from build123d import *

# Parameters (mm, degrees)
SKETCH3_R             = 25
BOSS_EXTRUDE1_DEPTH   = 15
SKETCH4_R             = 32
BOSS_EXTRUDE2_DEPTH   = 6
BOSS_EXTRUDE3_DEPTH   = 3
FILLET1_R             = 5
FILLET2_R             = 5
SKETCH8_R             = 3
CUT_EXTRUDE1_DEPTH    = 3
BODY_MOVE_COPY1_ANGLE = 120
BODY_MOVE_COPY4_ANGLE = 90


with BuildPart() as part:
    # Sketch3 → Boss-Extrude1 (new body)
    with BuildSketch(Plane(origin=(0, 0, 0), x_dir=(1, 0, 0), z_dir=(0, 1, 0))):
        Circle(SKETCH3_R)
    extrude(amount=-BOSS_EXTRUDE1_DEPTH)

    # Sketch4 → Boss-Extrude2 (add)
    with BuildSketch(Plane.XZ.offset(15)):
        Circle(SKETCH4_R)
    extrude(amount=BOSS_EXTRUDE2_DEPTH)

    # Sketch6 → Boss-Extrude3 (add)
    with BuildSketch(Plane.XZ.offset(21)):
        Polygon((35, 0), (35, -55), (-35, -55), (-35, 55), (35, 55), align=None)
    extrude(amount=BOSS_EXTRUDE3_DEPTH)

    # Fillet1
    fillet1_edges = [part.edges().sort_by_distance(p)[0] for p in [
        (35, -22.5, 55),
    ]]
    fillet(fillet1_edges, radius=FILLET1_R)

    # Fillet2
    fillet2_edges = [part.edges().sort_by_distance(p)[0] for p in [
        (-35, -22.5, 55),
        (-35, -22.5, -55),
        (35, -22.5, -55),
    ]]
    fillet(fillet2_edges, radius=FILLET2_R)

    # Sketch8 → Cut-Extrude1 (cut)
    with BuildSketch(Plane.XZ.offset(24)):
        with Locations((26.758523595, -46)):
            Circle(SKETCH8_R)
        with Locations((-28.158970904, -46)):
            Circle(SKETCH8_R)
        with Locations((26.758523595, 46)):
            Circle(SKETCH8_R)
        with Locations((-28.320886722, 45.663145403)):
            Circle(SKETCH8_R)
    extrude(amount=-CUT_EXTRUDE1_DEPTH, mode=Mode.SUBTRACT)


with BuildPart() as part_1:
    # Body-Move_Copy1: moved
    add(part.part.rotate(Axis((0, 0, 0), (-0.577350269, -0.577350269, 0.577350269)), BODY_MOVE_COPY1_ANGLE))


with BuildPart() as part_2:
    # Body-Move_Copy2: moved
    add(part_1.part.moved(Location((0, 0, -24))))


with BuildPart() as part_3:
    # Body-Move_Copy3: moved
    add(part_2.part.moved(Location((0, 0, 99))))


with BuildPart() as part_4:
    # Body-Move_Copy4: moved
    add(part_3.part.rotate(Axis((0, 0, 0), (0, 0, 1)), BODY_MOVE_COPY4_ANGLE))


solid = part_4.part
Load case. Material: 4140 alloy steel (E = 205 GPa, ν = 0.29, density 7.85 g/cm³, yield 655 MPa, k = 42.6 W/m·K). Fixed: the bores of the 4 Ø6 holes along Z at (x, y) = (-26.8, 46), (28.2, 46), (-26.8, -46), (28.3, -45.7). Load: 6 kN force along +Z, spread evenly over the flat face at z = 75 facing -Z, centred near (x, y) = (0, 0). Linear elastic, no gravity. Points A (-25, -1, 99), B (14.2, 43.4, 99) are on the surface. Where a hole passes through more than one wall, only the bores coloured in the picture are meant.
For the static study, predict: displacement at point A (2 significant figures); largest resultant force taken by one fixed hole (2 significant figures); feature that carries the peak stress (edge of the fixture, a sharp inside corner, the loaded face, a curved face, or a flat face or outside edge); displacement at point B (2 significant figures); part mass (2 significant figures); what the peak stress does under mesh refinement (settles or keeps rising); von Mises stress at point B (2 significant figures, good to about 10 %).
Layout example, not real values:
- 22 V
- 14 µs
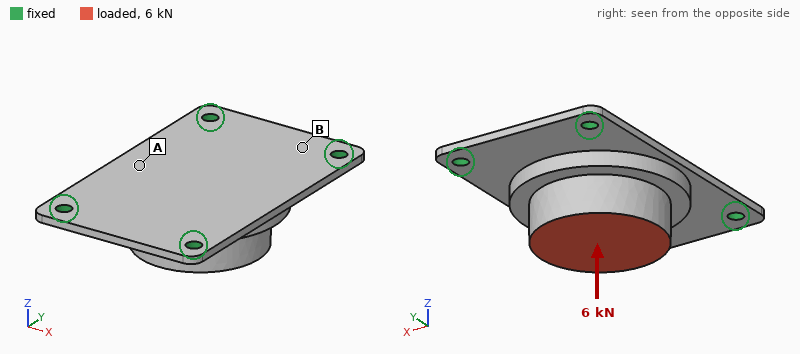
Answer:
- 0.12 mm
- 1.9 kN
- edge of the fixture
- 0.045 mm
- 560 g
- keeps rising
- 94 MPa
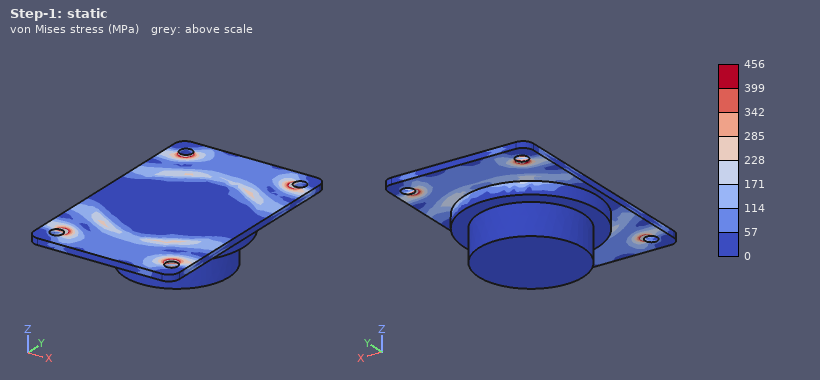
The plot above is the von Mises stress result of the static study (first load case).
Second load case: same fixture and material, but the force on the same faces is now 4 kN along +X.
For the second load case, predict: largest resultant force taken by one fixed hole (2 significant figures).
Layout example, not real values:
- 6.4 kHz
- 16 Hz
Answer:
- 1.7 kN
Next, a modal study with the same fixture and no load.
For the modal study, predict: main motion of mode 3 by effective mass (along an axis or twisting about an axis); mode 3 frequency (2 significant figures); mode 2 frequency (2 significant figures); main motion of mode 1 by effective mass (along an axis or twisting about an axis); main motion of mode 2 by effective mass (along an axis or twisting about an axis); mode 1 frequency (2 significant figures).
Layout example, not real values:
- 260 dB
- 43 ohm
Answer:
- along Y
- 3200 Hz
- 2000 Hz
- along Z
- along X
- 1600 Hz
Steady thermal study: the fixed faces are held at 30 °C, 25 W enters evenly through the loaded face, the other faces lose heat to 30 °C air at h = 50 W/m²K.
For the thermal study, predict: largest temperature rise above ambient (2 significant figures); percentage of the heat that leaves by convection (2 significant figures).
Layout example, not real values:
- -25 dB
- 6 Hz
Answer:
- 29 K
- 56 %
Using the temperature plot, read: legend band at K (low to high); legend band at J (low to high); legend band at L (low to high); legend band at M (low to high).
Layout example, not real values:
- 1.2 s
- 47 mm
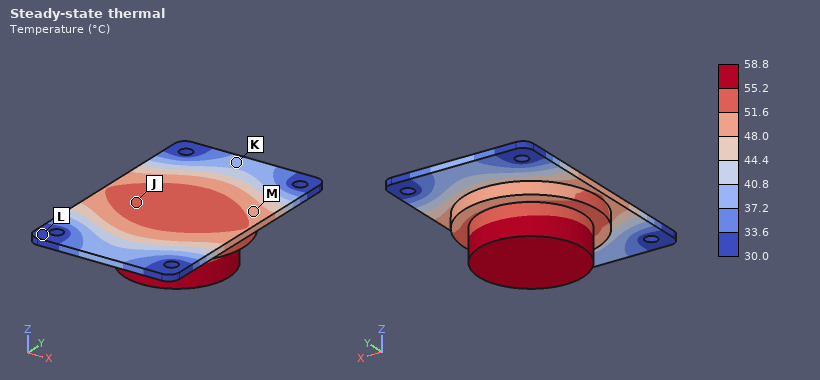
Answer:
- 37.2 to 40.8 °C
- 51.6 to 55.2 °C
- 30.0 to 33.6 °C
- 48.0 to 51.6 °C
